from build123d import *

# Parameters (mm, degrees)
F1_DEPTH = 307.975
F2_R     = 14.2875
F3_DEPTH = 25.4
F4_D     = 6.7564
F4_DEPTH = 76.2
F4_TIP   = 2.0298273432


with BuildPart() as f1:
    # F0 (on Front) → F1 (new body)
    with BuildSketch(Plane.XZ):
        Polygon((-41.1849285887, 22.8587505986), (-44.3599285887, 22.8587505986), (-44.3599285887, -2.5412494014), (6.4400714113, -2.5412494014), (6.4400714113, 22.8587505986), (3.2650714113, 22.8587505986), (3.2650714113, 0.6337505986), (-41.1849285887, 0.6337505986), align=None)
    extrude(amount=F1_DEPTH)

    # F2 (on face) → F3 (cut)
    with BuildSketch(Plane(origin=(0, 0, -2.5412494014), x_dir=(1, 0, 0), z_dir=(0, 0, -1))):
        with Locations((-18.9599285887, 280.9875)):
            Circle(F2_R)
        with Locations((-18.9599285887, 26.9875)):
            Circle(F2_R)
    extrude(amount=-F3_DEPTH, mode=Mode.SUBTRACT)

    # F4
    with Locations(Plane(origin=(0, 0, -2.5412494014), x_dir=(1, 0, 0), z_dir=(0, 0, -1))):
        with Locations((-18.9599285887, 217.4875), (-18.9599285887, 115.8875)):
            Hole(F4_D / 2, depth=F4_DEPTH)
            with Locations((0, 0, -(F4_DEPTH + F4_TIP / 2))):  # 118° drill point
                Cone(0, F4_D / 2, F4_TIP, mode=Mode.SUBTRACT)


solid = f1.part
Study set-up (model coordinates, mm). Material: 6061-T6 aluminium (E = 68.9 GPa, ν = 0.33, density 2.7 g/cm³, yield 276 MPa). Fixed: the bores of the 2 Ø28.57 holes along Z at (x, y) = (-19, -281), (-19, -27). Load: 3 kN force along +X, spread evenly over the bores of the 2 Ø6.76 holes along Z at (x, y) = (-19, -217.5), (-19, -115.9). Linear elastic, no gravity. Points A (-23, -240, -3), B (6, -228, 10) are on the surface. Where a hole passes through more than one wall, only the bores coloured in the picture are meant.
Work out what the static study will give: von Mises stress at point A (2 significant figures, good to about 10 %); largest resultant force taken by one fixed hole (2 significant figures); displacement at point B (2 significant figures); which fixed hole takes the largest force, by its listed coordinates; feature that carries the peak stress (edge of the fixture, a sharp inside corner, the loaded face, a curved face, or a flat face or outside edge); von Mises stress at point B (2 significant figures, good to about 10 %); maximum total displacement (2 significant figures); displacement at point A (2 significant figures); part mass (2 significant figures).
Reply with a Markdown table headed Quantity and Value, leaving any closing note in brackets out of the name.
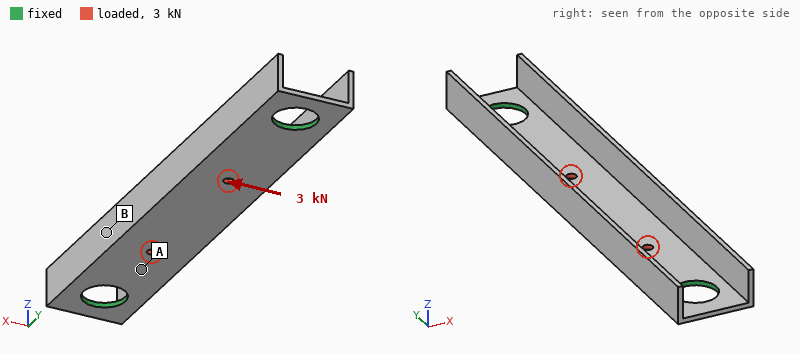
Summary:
| Quantity | Value |
|---|---|
| von Mises stress at point A | 18 MPa |
| largest resultant force taken by one fixed hole | 1.7 kN |
| displacement at point B | 0.064 mm |
| which fixed hole takes the largest force, by its listed coordinates | (-19, -281) |
| feature that carries the peak stress | edge of the fixture |
| von Mises stress at point B | 5.4 MPa |
| maximum total displacement | 0.15 mm |
| displacement at point A | 0.027 mm |
| part mass | 240 g |
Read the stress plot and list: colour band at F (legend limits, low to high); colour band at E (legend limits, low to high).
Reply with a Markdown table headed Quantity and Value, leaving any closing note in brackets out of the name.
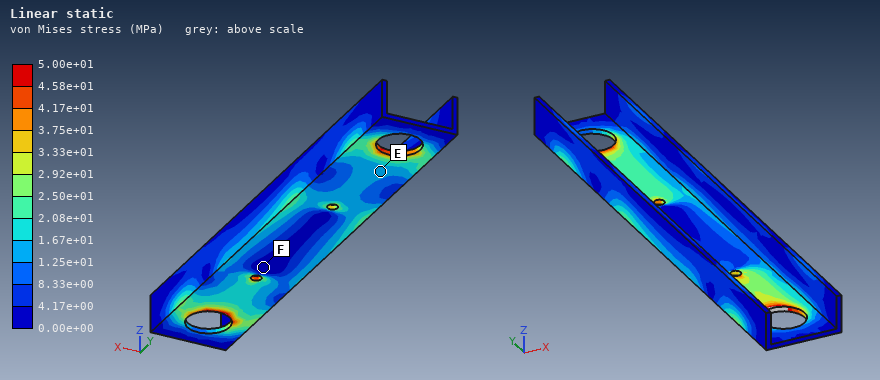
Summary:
| Quantity | Value |
|---|---|
| colour band at F | 0.00e+00 to 4.17e+00 MPa |
| colour band at E | 1.25e+01 to 1.67e+01 MPa |
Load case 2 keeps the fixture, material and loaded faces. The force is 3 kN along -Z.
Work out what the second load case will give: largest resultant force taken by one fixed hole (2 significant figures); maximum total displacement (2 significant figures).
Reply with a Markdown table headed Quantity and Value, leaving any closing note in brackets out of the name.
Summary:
| Quantity | Value |
|---|---|
| largest resultant force taken by one fixed hole | 3.5 kN |
| maximum total displacement | 0.61 mm |
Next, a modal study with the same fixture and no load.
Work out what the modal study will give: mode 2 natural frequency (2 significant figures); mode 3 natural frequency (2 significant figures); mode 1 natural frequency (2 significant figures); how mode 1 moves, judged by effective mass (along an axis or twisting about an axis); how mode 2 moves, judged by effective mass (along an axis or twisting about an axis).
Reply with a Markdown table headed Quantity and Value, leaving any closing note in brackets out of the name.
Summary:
| Quantity | Value |
|---|---|
| mode 2 natural frequency | 1200 Hz |
| mode 3 natural frequency | 2200 Hz |
| mode 1 natural frequency | 1200 Hz |
| how mode 1 moves, judged by effective mass | along X |
| how mode 2 moves, judged by effective mass | along Z |
